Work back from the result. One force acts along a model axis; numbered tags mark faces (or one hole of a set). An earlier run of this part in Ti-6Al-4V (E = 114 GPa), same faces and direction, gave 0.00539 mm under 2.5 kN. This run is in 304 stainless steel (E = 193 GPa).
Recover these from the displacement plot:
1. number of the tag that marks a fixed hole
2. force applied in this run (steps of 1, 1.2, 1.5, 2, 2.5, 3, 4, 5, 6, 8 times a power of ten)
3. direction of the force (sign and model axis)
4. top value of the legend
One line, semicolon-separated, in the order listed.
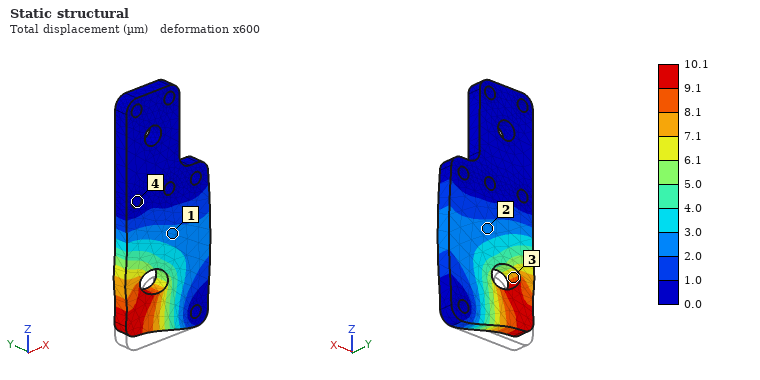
4; 8 kN; +Z; 10.1 µm
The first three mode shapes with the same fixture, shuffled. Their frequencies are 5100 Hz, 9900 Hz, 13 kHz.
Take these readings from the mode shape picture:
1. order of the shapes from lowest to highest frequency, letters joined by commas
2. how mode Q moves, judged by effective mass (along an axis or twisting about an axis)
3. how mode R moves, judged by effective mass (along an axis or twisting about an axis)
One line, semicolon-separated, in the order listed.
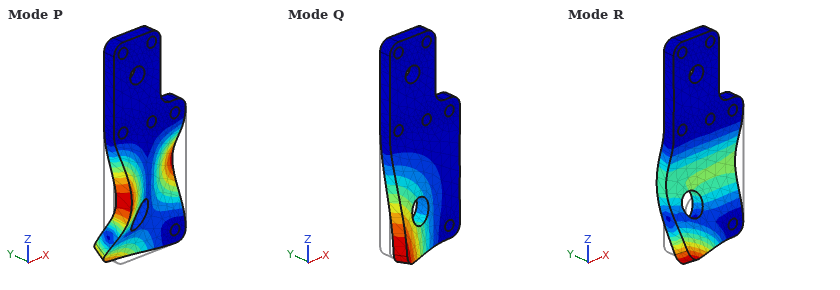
Q, R, P; along Y; along Y
